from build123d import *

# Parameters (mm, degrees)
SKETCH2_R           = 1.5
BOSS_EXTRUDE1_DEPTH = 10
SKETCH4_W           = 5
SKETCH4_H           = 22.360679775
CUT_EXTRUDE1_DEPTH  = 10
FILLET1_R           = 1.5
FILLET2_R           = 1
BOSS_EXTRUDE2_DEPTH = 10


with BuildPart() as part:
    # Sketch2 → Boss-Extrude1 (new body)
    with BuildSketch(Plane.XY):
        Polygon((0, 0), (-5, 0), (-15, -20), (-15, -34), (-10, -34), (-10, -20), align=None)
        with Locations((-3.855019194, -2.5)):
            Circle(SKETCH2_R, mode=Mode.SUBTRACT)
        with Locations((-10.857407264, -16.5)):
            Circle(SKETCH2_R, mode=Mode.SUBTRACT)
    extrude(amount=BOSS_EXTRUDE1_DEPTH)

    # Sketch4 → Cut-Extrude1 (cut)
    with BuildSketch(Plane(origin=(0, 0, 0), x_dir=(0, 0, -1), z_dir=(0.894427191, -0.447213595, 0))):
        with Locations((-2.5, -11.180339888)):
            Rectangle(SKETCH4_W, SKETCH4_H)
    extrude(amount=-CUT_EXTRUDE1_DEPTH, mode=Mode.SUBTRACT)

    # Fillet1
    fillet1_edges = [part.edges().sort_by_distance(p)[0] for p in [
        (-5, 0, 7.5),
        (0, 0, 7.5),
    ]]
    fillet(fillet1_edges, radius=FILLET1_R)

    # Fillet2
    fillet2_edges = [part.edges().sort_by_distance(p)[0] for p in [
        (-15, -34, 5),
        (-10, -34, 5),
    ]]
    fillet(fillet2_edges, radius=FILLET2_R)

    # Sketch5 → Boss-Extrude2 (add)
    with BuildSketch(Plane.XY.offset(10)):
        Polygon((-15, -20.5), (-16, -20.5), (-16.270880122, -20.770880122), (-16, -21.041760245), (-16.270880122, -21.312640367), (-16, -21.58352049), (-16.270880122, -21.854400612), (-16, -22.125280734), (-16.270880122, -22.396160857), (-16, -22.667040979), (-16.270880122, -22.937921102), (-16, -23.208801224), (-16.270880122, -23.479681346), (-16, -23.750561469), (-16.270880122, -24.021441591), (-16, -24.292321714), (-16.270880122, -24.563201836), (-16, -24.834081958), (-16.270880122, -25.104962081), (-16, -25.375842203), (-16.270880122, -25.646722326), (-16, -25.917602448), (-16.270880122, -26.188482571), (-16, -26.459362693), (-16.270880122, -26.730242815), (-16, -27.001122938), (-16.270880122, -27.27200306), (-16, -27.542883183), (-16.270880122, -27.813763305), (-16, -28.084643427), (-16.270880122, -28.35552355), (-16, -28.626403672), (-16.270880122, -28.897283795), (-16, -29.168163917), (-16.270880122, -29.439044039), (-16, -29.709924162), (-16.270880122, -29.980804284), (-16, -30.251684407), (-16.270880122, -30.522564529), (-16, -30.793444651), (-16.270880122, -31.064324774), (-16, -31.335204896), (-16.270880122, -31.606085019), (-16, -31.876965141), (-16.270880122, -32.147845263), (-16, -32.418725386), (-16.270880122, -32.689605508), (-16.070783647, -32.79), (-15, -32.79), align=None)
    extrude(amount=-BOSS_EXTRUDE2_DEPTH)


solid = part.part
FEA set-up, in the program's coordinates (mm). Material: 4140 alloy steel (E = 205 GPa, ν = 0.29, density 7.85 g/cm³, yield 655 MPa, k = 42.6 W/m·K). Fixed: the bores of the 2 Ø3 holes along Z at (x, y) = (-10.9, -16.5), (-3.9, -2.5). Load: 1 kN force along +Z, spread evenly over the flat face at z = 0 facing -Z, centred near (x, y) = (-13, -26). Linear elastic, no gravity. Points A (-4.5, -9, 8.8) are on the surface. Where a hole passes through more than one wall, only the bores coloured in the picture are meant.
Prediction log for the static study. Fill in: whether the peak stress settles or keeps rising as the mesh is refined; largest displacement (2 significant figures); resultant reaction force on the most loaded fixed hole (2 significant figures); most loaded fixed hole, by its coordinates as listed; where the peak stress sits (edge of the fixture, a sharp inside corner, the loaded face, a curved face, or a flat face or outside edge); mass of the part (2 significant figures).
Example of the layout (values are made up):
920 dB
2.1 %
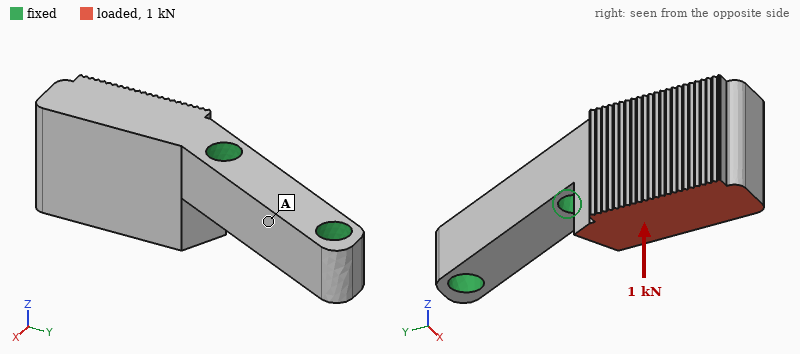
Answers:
keeps rising
56 µm
1.0 kN
(-10.9, -16.5)
edge of the fixture
10 g
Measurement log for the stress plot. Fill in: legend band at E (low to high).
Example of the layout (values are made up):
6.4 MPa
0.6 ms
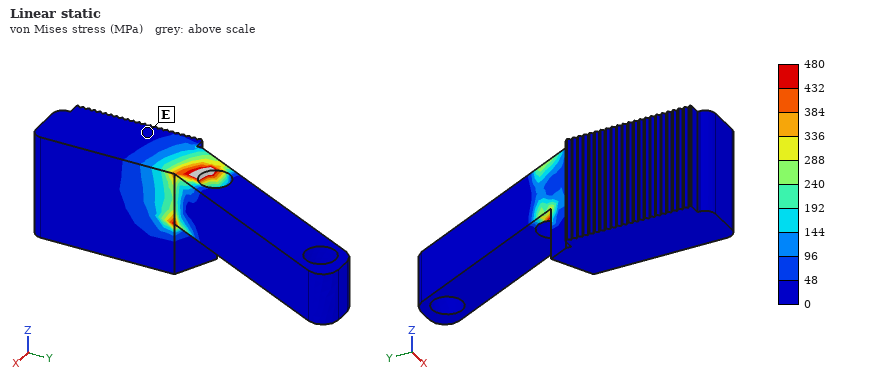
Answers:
0 to 48 MPa
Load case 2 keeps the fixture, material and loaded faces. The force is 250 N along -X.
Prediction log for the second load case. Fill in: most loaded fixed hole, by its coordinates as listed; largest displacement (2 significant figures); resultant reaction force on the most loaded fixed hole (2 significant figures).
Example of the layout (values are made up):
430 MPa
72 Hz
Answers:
(-10.9, -16.5)
27 µm
250 N
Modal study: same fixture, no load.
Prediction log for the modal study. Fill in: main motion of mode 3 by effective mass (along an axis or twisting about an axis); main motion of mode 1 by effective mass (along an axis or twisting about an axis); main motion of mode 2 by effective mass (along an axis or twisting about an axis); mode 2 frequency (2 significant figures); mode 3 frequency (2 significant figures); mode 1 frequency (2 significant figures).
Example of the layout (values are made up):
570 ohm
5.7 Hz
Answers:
twisting about Y
along X
along Z
9700 Hz
21 kHz
8300 Hz
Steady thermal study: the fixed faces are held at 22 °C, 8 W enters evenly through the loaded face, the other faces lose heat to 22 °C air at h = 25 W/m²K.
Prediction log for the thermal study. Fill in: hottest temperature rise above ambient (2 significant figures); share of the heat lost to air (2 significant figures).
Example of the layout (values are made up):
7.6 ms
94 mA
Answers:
54 K
6.6 %
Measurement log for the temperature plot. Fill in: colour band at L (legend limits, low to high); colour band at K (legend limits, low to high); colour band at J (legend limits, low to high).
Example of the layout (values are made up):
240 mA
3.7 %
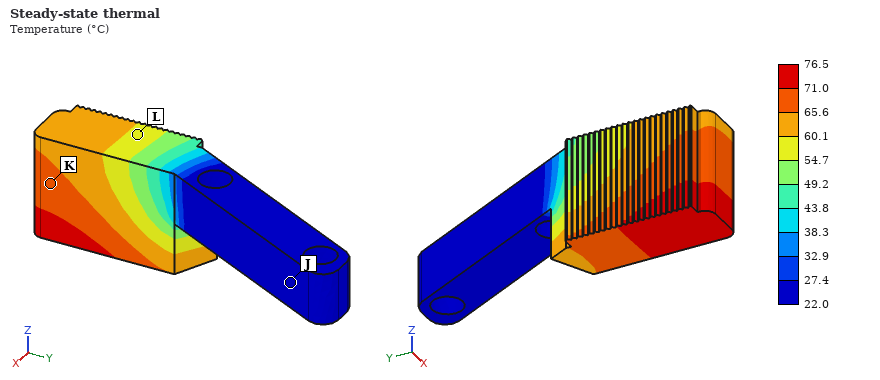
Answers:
54.7 to 60.1 °C
65.6 to 71.0 °C
22.0 to 27.4 °C
